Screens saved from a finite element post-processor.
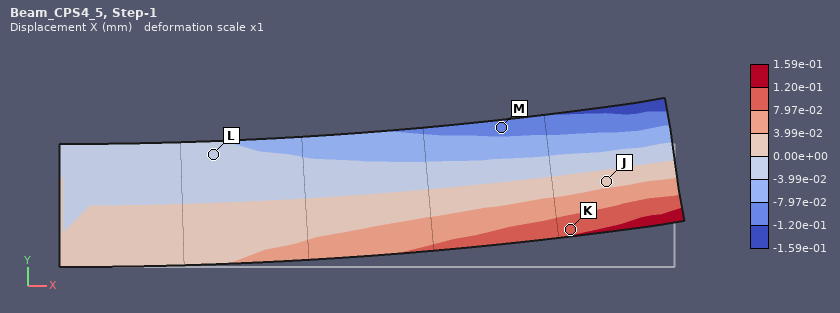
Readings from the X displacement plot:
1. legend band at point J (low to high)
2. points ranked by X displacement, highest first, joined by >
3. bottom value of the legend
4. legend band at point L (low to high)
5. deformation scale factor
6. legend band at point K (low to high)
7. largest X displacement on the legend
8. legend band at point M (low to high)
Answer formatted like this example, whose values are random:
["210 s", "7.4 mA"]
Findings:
["0.00e+00 to 3.99e-02 mm", "K > J > L > M", "-1.59e-01 mm", "-3.99e-02 to 0.00e+00 mm", "1", "7.97e-02 to 1.20e-01 mm", "1.59e-01 mm", "-1.20e-01 to -7.97e-02 mm"]
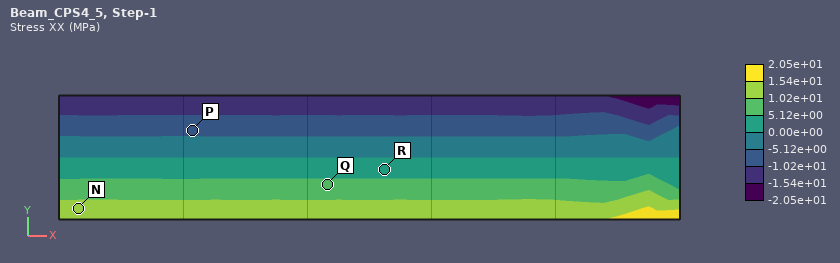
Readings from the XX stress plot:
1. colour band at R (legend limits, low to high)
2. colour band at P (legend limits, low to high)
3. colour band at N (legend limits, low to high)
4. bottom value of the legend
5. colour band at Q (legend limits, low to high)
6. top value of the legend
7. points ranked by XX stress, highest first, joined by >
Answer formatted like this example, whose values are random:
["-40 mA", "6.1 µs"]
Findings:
["0.00e+00 to 5.12e+00 MPa", "-1.02e+01 to -5.12e+00 MPa", "1.02e+01 to 1.54e+01 MPa", "-2.05e+01 MPa", "5.12e+00 to 1.02e+01 MPa", "2.05e+01 MPa", "N > Q > R > P"]
